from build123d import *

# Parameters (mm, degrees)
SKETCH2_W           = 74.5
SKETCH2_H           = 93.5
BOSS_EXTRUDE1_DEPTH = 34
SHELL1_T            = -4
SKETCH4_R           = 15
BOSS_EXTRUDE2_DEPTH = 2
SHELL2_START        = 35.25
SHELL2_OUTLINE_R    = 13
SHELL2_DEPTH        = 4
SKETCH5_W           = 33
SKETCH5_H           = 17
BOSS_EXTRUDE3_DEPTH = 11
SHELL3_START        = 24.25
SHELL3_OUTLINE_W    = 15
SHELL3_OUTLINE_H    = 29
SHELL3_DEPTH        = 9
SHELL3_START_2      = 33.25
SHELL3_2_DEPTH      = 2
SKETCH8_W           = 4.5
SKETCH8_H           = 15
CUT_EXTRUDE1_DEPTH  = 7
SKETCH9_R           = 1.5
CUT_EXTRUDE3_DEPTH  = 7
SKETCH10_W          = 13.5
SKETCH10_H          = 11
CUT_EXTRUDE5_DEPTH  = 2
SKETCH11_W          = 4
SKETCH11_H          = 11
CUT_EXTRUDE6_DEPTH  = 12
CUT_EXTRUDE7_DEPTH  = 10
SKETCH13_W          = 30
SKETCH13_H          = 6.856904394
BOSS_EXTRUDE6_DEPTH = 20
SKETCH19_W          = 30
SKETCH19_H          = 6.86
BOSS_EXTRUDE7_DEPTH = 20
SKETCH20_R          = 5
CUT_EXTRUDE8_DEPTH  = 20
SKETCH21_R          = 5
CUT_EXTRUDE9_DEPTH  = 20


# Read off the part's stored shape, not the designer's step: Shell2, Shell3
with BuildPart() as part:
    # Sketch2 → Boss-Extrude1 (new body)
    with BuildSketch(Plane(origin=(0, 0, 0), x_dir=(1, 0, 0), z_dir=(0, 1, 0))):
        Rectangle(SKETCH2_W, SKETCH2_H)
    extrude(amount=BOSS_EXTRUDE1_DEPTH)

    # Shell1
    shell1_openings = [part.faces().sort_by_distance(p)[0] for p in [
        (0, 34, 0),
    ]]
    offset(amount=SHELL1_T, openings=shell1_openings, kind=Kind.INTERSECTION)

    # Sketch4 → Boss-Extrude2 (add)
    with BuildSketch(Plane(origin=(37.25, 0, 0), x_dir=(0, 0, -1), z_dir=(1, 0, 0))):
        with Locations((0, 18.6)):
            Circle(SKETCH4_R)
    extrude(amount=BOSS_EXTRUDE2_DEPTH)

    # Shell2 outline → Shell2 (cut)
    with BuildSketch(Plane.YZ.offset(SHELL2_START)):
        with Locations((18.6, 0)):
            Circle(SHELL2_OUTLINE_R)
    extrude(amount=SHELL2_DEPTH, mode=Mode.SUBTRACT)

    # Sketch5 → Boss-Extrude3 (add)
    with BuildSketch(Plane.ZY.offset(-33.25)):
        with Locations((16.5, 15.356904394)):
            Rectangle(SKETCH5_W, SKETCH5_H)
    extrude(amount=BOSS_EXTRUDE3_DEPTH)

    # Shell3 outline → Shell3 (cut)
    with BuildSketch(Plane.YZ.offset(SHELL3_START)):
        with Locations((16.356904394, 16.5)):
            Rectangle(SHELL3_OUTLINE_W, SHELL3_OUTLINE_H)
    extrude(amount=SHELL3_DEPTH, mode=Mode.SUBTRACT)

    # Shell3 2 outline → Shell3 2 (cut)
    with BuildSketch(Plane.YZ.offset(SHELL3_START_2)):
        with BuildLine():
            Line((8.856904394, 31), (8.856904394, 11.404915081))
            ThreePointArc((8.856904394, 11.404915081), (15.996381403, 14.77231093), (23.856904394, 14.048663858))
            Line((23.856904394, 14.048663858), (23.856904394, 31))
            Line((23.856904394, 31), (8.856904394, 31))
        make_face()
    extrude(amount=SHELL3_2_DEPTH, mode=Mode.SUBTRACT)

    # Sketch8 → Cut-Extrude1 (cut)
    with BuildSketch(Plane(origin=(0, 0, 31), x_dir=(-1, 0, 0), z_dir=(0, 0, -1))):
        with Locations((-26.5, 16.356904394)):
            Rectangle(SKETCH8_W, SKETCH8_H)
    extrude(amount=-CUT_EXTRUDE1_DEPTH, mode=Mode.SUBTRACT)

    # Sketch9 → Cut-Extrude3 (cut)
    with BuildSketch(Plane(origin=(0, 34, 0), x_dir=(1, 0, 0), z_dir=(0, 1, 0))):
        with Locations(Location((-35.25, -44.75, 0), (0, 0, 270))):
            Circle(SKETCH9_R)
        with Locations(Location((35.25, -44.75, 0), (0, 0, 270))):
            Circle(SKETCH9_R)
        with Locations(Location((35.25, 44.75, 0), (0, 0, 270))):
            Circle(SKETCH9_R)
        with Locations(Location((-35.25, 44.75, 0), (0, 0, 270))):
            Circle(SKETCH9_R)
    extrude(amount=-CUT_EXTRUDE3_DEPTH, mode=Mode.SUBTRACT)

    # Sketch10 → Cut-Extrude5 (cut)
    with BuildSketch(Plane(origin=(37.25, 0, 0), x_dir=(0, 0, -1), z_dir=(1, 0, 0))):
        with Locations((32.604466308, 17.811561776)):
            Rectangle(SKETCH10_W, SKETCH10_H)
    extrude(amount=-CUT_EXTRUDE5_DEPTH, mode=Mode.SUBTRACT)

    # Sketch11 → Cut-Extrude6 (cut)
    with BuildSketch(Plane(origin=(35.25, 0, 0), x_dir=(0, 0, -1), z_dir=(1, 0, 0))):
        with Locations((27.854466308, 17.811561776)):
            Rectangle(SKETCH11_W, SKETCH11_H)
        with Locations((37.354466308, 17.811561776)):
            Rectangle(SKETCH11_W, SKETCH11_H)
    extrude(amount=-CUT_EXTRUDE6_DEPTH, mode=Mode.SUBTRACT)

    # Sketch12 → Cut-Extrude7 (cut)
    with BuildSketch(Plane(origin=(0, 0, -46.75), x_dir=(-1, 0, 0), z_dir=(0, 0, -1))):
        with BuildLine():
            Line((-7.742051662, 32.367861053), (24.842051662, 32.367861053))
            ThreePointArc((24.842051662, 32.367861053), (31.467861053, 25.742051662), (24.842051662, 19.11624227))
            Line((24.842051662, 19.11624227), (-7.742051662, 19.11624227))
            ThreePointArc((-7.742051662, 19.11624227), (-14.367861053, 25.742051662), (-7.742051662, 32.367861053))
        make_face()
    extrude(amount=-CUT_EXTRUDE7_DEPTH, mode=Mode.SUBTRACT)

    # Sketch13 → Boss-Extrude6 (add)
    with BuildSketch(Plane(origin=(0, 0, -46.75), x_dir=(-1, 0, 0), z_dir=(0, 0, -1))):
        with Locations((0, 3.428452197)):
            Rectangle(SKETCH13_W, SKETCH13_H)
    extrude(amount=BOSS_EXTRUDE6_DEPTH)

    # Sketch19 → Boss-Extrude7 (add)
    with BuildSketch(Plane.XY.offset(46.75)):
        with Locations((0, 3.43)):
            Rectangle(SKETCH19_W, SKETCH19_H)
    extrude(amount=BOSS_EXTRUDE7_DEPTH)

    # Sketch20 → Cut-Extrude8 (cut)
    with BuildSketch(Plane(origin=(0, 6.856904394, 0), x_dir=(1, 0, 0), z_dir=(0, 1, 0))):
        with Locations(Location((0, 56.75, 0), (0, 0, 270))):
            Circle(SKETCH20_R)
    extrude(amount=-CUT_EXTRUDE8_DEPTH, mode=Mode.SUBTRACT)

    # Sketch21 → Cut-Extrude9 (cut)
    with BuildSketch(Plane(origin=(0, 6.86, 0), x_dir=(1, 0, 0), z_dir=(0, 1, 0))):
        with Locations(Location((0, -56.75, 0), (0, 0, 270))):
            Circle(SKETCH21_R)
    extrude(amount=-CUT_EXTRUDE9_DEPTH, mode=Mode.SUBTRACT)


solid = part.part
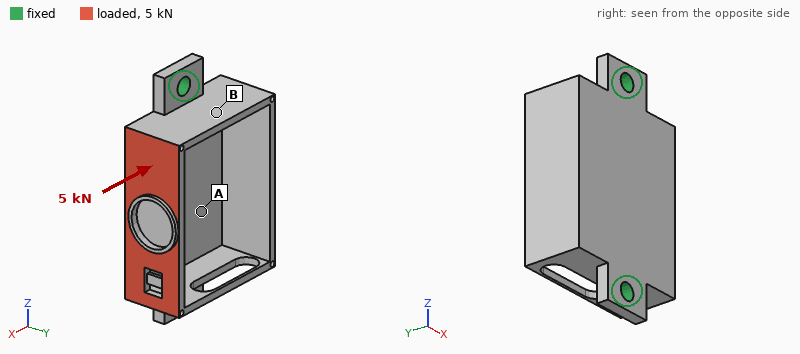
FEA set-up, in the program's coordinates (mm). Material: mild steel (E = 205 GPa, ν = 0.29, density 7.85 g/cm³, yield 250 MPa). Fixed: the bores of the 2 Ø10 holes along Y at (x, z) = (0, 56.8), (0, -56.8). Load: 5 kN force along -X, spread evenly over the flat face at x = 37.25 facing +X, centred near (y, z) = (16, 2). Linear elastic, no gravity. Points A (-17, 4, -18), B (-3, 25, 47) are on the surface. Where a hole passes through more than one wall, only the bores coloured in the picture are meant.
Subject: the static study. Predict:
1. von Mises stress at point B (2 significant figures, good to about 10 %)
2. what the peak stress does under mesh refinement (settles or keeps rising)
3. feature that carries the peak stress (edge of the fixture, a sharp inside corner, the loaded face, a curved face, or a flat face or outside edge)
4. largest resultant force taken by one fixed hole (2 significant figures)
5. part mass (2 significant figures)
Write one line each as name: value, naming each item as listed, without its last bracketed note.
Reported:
von Mises stress at point B: 28 MPa
what the peak stress does under mesh refinement: keeps rising
feature that carries the peak stress: a sharp inside corner
largest resultant force taken by one fixed hole: 2.6 kN
part mass: 560 g
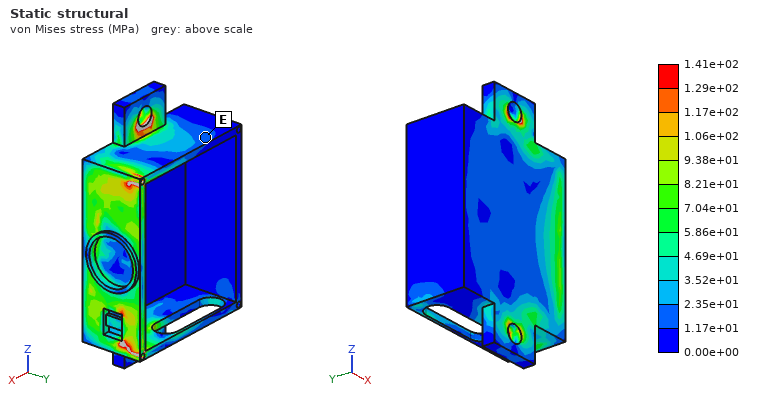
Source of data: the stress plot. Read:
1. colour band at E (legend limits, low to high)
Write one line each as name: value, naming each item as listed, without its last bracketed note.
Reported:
colour band at E: 1.17e+01 to 2.35e+01 MPa
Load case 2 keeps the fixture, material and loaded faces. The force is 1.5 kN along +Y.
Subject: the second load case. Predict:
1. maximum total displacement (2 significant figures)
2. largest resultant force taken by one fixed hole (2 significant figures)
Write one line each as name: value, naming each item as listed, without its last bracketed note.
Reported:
maximum total displacement: 66 µm
largest resultant force taken by one fixed hole: 790 N
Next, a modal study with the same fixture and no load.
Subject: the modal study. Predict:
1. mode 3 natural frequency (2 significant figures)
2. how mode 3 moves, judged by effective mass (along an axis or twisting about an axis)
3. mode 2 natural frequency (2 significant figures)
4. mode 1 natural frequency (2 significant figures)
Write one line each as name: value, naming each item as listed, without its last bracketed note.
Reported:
mode 3 natural frequency: 3100 Hz
how mode 3 moves, judged by effective mass: along Y
mode 2 natural frequency: 2900 Hz
mode 1 natural frequency: 1800 Hz
